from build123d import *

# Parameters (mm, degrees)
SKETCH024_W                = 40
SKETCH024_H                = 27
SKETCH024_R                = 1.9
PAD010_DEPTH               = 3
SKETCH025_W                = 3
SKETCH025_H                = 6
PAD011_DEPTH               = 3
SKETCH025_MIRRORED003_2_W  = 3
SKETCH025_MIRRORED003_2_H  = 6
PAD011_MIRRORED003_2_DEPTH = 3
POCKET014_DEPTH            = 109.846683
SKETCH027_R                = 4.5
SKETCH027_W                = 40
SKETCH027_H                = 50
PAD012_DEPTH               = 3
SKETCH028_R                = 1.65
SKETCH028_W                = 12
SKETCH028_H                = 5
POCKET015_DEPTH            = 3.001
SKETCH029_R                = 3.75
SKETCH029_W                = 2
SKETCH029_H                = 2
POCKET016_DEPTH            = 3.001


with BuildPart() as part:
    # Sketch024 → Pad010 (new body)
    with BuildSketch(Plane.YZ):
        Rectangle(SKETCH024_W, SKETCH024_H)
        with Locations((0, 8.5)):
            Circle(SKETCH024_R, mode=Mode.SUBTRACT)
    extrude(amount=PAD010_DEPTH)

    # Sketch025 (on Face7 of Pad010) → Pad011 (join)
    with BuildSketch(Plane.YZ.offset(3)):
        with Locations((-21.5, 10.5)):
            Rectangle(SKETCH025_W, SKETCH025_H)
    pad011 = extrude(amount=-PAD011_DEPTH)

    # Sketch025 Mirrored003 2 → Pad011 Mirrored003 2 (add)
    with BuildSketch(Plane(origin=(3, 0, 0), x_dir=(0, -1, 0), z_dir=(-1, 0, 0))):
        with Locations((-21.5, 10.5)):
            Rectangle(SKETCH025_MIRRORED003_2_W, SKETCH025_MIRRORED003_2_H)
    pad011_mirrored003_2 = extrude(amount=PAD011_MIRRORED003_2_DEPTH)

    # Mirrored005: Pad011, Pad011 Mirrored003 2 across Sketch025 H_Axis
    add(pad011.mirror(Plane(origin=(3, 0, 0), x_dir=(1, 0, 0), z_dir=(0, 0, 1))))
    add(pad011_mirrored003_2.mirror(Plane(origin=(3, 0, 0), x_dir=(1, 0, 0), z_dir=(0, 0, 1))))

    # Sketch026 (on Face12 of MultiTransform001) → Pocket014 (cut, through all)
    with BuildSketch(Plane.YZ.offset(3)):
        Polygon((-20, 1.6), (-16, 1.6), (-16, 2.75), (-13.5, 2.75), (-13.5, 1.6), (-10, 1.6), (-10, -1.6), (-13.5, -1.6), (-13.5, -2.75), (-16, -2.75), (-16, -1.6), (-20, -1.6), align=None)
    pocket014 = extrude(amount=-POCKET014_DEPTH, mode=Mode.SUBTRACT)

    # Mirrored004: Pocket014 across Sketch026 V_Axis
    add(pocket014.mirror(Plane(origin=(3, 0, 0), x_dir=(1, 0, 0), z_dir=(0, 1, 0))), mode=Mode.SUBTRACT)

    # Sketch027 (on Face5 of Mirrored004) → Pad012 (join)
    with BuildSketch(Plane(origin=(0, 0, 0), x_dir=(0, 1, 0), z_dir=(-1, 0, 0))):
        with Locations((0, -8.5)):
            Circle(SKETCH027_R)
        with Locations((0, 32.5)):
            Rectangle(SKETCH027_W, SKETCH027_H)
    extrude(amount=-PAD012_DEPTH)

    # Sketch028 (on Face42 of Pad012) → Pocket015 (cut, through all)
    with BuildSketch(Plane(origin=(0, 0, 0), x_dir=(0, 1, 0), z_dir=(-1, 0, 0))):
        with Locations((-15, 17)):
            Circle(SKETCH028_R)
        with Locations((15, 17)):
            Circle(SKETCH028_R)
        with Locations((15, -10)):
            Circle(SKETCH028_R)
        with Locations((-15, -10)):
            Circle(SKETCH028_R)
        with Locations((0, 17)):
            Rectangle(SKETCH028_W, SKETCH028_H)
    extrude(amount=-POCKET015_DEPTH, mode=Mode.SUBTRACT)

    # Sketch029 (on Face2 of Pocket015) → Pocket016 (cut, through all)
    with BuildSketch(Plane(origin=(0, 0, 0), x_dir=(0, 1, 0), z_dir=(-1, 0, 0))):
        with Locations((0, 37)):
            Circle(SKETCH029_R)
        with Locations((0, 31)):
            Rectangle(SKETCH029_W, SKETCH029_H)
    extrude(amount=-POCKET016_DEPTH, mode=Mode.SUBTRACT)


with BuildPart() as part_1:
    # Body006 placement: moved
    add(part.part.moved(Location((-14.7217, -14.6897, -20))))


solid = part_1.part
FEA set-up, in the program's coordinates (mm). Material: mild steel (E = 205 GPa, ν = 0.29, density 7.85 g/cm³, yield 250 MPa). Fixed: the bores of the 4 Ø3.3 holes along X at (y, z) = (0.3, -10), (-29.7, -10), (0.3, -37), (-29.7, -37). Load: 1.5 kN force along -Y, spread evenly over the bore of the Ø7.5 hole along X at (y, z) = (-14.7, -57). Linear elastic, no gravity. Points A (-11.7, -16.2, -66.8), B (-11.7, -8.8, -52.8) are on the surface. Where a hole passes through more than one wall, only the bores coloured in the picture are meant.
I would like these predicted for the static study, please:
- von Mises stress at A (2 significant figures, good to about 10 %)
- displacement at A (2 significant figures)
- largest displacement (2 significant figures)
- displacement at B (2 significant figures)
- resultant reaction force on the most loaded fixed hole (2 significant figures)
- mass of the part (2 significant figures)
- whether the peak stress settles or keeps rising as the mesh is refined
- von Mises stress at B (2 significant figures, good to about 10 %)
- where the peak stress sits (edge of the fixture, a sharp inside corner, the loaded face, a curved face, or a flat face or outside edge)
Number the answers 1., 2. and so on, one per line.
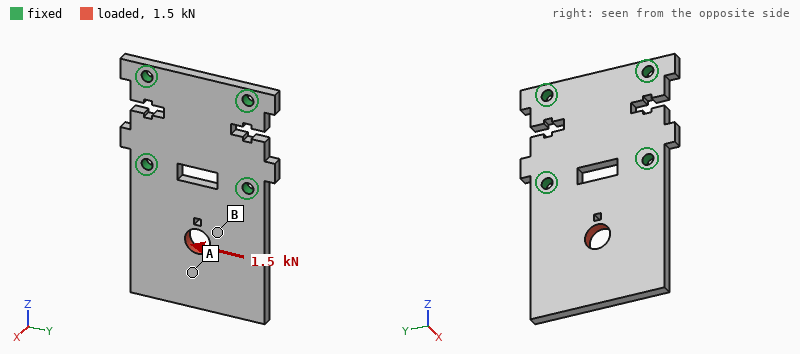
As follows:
1. 9.4 MPa
2. 7.5 µm
3. 8.9 µm
4. 4.7 µm
5. 1.2 kN
6. 63 g
7. keeps rising
8. 29 MPa
9. edge of the fixture
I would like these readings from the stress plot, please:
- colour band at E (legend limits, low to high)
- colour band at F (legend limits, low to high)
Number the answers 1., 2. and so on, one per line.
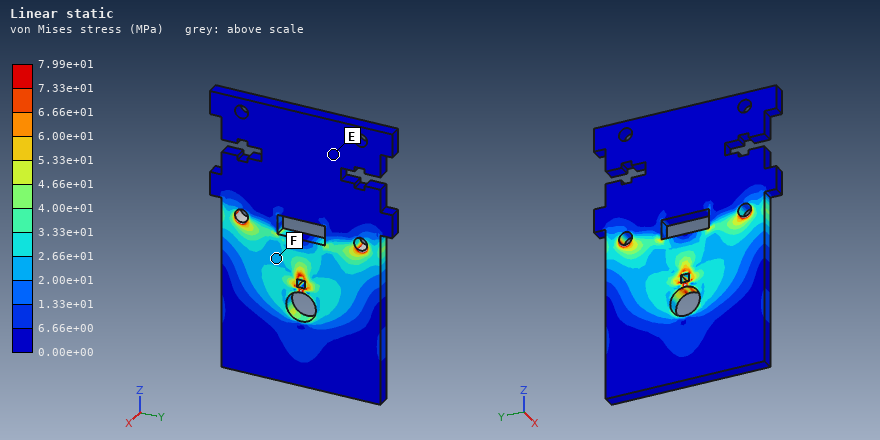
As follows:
1. 0.00e+00 to 6.66e+00 MPa
2. 2.00e+01 to 2.66e+01 MPa
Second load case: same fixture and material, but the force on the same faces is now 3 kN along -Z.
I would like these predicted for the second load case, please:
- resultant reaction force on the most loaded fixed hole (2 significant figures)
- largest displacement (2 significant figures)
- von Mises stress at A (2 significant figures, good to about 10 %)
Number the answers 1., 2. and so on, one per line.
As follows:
1. 1.4 kN
2. 5.6 µm
3. 21 MPa
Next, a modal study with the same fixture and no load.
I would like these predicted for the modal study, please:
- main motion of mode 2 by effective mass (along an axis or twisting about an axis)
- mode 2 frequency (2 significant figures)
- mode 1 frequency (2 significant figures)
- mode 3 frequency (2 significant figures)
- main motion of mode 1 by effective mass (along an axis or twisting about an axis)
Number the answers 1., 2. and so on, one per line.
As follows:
1. twisting about Z
2. 3700 Hz
3. 1400 Hz
4. 8600 Hz
5. along X
